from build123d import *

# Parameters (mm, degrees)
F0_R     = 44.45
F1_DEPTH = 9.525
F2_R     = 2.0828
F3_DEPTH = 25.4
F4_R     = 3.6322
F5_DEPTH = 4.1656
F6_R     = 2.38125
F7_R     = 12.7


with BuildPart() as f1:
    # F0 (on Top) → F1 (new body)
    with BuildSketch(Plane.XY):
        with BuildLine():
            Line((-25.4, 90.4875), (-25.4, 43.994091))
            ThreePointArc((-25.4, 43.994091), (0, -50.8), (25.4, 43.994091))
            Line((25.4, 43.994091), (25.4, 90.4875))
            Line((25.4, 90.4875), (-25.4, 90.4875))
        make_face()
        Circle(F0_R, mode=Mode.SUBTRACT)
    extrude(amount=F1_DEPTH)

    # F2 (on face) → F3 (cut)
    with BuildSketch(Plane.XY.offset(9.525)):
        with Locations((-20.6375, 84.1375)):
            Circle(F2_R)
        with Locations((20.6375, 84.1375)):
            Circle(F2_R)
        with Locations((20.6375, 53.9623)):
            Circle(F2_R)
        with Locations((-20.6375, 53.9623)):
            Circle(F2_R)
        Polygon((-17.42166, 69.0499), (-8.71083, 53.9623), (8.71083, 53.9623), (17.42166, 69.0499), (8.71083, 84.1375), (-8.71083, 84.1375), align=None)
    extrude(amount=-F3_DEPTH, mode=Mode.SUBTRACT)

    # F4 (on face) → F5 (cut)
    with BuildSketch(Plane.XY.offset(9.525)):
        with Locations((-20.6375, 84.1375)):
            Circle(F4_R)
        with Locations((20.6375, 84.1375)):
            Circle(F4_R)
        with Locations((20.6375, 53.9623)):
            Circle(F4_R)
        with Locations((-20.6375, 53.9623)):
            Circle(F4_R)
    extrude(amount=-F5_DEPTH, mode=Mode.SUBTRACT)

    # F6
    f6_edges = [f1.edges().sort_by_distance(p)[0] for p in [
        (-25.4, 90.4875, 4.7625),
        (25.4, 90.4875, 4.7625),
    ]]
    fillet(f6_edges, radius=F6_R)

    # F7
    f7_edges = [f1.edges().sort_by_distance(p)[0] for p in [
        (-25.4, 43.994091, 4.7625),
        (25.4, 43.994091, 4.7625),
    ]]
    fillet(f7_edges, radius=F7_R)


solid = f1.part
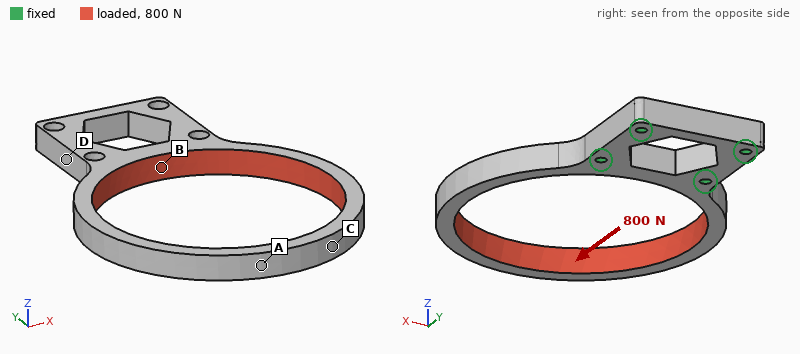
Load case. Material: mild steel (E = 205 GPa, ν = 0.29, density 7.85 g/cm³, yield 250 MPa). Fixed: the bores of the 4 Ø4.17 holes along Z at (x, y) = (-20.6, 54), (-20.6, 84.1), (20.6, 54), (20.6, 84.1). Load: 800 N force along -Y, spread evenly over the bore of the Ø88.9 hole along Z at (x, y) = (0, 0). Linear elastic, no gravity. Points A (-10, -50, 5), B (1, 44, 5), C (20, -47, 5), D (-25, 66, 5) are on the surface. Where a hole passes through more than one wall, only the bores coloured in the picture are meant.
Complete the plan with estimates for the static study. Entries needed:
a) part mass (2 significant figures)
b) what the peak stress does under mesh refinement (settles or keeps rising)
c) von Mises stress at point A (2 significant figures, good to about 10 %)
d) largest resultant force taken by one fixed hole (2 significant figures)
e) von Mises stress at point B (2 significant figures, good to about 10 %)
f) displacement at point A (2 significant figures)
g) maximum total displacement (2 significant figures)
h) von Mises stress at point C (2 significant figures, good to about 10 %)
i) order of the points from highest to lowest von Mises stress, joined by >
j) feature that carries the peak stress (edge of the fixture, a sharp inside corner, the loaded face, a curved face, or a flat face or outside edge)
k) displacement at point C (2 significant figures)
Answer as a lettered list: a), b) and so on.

a) 240 g
b) keeps rising
c) 25 MPa
d) 470 N
e) 9.2 MPa
f) 55 µm
g) 58 µm
h) 19 MPa
i) A > C > B > D
j) edge of the fixture
k) 49 µm
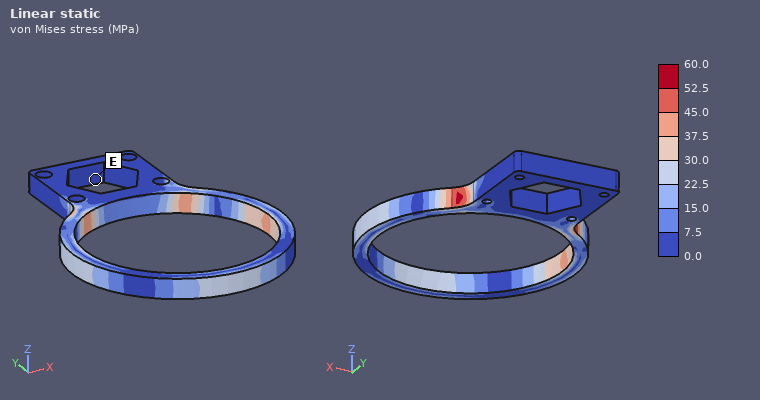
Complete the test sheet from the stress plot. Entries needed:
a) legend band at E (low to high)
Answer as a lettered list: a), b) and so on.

a) 0.0 to 7.5 MPa
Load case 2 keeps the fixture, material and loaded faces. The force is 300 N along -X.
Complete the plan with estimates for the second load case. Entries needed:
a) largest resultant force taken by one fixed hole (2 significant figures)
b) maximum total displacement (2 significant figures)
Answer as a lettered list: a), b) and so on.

a) 330 N
b) 0.16 mm
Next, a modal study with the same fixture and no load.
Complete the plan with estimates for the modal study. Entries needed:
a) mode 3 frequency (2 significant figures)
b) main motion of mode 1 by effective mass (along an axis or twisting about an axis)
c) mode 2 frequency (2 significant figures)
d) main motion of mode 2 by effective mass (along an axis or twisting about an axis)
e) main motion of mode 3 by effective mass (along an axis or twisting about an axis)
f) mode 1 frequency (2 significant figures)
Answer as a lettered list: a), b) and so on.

a) 1200 Hz
b) along Z
c) 620 Hz
d) along X
e) twisting about Y
f) 460 Hz
